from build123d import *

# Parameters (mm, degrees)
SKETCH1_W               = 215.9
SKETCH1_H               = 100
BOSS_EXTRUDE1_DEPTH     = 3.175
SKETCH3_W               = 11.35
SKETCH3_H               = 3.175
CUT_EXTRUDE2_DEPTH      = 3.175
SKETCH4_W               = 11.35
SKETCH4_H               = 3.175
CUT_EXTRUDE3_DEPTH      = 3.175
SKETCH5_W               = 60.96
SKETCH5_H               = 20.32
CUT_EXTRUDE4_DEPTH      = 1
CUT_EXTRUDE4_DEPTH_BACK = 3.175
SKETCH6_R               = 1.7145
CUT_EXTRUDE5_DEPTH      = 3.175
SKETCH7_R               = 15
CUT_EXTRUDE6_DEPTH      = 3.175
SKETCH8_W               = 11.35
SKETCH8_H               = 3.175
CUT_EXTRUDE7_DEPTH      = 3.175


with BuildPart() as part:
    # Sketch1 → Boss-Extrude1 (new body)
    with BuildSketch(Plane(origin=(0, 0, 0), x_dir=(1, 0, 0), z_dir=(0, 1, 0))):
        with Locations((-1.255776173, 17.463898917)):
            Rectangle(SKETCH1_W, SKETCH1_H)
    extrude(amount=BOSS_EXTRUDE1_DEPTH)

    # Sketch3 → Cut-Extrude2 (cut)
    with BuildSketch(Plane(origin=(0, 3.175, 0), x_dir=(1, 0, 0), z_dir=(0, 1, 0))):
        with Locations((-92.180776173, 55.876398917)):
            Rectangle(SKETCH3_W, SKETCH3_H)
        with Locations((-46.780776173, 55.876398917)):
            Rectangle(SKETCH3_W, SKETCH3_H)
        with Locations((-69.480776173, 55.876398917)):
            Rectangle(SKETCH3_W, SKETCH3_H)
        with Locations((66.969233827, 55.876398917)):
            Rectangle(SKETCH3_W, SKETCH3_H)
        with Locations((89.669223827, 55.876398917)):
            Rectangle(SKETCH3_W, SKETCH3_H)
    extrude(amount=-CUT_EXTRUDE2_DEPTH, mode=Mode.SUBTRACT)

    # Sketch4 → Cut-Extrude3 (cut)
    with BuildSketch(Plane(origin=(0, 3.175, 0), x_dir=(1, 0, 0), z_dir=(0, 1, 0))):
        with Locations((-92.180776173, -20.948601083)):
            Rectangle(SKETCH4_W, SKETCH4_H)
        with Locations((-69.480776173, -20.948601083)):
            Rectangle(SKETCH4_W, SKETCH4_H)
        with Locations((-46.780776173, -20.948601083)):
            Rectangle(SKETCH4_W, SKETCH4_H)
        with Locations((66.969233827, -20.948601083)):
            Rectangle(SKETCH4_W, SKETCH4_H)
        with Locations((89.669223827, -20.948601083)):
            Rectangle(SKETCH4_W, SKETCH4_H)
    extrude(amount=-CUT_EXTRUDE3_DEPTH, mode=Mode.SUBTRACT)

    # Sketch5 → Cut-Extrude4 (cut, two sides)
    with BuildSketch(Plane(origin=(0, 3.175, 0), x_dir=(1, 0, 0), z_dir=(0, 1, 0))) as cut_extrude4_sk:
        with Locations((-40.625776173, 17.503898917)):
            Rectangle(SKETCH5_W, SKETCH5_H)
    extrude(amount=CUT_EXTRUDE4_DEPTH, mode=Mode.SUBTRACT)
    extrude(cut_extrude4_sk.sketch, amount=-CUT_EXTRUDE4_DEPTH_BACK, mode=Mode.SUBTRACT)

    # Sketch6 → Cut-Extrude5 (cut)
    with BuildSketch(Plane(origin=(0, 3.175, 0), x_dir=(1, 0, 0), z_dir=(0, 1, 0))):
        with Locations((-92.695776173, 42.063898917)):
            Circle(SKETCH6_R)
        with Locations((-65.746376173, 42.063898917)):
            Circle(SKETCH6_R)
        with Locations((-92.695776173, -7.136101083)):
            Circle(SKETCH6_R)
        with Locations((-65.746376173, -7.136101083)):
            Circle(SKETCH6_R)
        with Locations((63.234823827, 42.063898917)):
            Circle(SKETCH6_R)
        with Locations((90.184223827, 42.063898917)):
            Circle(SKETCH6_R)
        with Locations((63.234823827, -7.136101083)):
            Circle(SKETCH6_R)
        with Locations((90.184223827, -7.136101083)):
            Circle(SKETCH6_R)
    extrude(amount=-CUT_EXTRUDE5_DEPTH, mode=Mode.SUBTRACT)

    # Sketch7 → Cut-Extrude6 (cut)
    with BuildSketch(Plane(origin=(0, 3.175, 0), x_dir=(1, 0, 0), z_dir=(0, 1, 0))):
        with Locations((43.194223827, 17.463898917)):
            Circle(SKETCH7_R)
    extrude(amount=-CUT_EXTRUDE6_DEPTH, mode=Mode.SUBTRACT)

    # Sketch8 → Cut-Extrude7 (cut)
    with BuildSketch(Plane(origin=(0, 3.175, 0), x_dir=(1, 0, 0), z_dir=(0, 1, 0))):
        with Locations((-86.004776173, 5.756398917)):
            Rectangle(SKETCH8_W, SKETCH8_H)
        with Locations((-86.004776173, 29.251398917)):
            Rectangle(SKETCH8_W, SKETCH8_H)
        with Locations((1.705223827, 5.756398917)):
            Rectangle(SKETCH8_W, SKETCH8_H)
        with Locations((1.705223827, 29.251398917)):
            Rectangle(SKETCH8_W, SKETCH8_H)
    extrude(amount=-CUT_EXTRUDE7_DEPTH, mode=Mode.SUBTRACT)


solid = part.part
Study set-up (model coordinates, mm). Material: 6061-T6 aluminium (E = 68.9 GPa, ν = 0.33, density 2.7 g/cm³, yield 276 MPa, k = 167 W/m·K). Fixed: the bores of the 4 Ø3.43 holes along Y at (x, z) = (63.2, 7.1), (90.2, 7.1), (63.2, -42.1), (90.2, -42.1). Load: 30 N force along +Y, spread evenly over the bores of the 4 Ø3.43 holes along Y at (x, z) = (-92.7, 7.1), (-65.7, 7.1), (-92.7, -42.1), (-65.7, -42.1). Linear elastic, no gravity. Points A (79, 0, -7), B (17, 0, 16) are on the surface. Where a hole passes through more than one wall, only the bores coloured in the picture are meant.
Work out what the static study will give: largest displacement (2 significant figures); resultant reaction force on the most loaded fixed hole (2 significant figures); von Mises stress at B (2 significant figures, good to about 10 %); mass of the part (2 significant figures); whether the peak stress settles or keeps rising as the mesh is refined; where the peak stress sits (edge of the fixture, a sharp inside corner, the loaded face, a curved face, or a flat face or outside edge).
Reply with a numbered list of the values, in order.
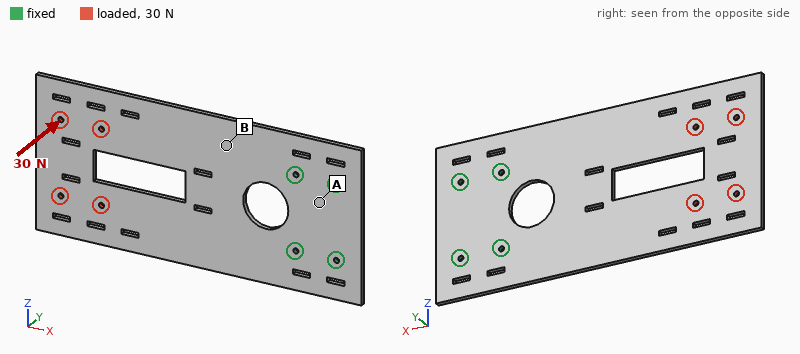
1. 2.7 mm
2. 51 N
3. 19 MPa
4. 160 g
5. keeps rising
6. edge of the fixture
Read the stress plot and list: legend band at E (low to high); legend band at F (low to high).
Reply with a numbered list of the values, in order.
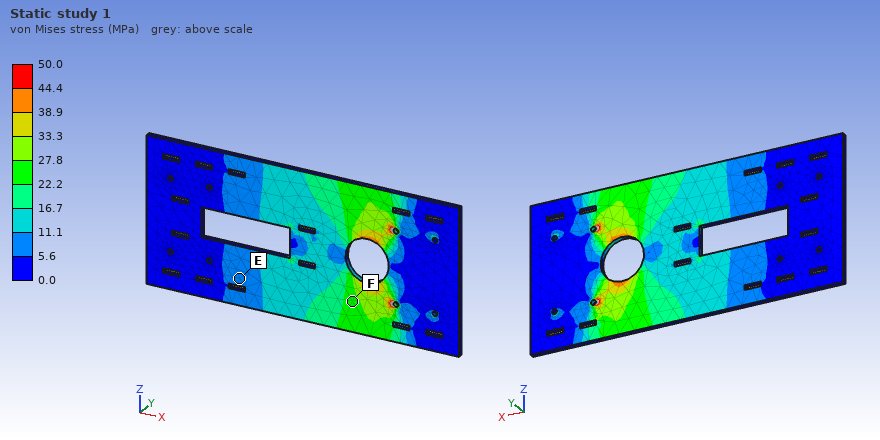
1. 5.6 to 11.1 MPa
2. 22.2 to 27.8 MPa
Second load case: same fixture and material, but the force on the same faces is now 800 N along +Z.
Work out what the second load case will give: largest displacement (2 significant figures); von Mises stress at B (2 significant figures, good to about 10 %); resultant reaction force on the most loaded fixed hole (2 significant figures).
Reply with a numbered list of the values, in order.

1. 0.15 mm
2. 9.2 MPa
3. 1.4 kN
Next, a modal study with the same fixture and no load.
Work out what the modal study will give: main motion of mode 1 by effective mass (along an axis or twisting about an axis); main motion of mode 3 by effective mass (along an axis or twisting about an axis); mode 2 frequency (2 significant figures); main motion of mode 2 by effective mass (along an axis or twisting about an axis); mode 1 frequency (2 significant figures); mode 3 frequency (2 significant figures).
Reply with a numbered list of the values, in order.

1. along Y
2. along Y
3. 300 Hz
4. twisting about X
5. 81 Hz
6. 500 Hz
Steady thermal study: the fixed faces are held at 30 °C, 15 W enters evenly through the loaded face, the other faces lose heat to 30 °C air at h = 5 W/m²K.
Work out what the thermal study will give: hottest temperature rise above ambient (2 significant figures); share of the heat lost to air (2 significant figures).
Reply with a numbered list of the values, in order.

1. 44 K
2. 28 %
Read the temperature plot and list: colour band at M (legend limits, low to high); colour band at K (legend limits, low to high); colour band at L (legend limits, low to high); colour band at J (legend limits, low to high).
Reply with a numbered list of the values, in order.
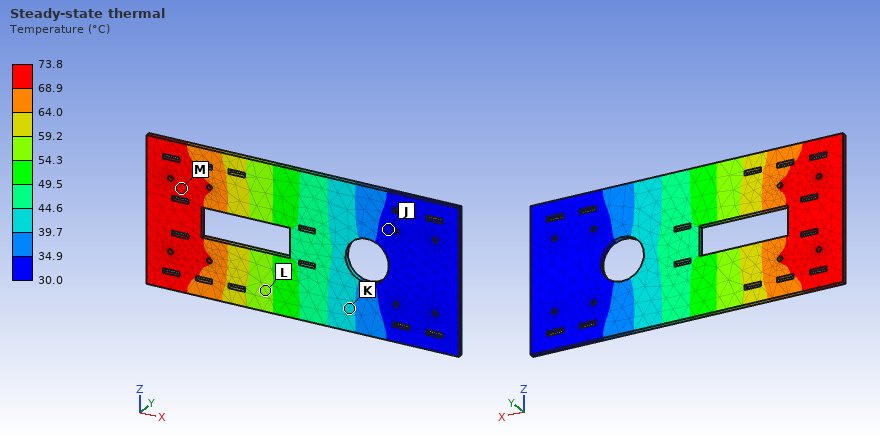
1. 68.9 to 73.8 °C
2. 39.7 to 44.6 °C
3. 54.3 to 59.2 °C
4. 30.0 to 34.9 °C
